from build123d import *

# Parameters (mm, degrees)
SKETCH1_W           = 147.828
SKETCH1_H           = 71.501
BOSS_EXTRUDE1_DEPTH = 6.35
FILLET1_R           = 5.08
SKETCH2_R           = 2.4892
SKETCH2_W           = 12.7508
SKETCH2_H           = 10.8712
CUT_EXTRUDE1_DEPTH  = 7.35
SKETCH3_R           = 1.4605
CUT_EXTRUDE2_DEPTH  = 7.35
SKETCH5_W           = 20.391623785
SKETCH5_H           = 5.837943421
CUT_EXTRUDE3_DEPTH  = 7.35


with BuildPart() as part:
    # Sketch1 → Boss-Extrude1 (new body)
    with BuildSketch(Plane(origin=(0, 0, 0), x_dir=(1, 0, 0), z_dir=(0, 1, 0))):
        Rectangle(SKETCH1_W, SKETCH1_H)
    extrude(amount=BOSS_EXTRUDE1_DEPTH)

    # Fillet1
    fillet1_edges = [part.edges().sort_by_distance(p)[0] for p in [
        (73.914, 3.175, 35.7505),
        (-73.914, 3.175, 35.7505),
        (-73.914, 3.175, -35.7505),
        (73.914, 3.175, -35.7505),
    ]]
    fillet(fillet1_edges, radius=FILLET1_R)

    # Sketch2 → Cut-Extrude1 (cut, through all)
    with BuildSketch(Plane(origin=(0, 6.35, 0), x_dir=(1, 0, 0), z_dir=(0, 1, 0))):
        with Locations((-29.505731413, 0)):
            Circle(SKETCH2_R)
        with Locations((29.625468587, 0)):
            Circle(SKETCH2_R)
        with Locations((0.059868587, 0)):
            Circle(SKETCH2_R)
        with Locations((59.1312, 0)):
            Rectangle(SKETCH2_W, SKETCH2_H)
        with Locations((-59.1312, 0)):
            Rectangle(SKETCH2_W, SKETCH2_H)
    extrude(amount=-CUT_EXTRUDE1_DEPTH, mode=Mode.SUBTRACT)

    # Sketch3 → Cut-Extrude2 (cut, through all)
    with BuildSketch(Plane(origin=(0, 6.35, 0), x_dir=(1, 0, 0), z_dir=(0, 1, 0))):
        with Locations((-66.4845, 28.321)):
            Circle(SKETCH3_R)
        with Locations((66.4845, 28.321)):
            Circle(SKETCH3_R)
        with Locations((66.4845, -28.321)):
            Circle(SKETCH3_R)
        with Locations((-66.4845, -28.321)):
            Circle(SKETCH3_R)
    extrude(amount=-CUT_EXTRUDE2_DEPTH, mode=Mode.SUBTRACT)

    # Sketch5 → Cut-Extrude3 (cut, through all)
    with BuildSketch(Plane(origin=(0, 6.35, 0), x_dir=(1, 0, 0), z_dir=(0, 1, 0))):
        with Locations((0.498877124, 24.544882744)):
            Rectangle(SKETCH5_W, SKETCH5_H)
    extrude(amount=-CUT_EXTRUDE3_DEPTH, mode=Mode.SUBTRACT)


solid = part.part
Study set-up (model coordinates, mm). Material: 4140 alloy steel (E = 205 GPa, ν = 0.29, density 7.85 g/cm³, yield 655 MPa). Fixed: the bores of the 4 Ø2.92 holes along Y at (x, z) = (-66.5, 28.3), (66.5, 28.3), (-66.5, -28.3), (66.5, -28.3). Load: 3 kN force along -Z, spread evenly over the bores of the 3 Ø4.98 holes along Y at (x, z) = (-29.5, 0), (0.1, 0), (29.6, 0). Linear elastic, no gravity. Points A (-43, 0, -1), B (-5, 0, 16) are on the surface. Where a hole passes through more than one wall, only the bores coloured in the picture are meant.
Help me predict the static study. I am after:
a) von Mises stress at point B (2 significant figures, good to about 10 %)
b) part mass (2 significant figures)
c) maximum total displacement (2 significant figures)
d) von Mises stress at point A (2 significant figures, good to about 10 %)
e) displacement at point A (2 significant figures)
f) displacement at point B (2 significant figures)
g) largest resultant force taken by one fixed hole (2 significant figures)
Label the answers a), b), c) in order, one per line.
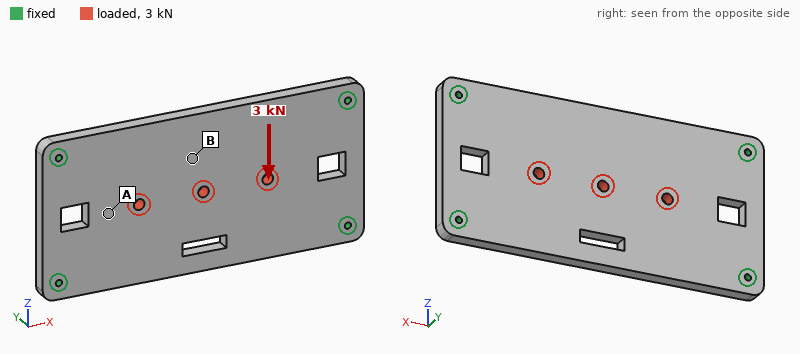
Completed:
a) 2.6 MPa
b) 500 g
c) 4.2 µm
d) 11 MPa
e) 2.1 µm
f) 3.8 µm
g) 1.1 kN
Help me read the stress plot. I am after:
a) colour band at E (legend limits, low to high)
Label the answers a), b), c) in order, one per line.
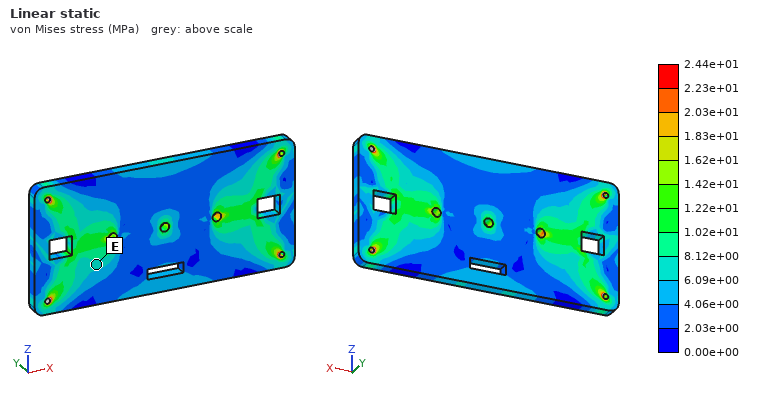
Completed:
a) 6.09e+00 to 8.12e+00 MPa
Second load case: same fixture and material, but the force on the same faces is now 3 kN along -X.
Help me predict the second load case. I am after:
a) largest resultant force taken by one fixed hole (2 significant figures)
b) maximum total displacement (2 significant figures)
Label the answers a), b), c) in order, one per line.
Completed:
a) 790 N
b) 1.8 µm
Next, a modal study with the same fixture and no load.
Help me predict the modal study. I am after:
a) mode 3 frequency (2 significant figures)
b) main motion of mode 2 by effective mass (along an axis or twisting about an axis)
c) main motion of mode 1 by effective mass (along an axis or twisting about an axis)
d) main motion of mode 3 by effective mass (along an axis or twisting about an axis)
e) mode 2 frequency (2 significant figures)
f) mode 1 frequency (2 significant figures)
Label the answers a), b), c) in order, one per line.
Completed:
a) 4300 Hz
b) twisting about X
c) along Y
d) twisting about Z
e) 2800 Hz
f) 1500 Hz
